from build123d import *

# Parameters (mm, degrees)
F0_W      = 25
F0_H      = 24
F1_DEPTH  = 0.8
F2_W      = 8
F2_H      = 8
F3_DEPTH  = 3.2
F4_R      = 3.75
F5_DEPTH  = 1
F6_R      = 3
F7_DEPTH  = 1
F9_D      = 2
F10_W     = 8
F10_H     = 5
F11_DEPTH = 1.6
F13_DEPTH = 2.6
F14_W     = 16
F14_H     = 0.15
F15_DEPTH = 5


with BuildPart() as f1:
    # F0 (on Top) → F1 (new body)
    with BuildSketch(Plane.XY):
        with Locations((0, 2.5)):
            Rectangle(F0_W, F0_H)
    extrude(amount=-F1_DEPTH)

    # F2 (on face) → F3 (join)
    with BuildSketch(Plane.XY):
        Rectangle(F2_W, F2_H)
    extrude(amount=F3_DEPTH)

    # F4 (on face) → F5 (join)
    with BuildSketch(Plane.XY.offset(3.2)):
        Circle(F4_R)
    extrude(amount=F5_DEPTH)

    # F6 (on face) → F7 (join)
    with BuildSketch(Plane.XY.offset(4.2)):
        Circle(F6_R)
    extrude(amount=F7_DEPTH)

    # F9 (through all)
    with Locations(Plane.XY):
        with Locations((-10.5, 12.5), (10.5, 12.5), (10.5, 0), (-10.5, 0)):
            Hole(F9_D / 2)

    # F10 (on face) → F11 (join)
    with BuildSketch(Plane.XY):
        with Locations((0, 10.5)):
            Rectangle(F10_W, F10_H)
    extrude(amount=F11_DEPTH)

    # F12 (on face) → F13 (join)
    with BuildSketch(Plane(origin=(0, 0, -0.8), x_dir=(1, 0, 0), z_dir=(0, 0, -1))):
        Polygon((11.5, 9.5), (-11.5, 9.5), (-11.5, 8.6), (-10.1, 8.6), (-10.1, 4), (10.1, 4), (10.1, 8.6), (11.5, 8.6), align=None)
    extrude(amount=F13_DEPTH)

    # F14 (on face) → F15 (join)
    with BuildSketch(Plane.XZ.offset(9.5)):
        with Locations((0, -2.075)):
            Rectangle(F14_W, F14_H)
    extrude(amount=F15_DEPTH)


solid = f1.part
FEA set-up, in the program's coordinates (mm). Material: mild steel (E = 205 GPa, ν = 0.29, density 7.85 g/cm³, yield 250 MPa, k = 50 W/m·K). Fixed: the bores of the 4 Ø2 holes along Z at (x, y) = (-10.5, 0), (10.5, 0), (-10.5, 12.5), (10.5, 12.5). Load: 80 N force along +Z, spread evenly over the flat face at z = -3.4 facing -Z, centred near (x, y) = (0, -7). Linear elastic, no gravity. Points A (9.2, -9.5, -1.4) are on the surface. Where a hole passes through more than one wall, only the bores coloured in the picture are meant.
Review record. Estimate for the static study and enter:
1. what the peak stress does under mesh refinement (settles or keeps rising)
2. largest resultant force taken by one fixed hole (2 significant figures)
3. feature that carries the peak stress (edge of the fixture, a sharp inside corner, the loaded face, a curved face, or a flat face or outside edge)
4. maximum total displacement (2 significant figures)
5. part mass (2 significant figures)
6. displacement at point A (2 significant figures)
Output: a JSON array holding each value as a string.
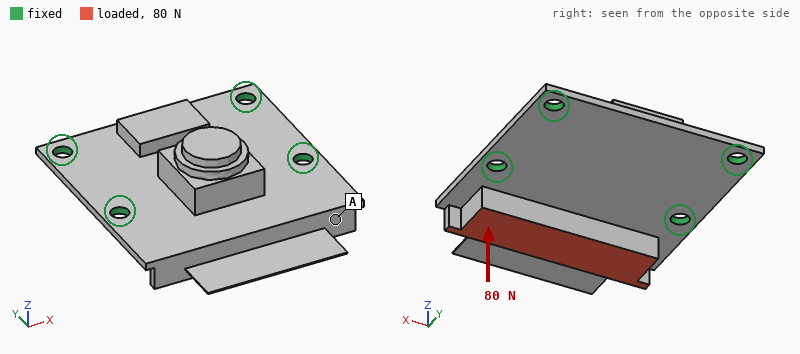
["keeps rising", "50 N", "edge of the fixture", "55 µm", "8.8 g", "34 µm"]
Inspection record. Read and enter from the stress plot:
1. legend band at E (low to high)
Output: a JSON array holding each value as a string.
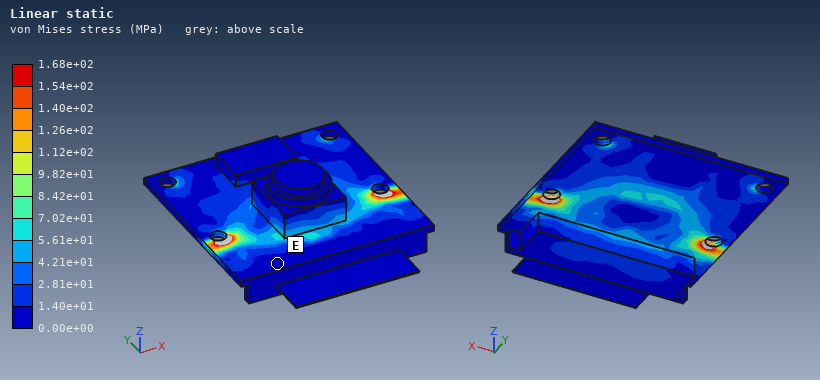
["0.00e+00 to 1.40e+01 MPa"]
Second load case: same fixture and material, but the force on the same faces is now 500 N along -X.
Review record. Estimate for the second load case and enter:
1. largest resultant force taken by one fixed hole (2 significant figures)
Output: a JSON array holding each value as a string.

["280 N"]
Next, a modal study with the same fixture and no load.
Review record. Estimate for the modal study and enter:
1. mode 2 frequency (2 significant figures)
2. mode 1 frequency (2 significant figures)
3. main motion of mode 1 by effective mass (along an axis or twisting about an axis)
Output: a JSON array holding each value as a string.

["5500 Hz", "4200 Hz", "along Z"]
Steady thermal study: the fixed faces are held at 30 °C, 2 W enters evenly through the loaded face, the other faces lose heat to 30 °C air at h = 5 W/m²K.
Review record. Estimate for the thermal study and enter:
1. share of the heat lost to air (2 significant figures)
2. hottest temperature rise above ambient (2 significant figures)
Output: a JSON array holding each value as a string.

["3.0 %", "14 K"]
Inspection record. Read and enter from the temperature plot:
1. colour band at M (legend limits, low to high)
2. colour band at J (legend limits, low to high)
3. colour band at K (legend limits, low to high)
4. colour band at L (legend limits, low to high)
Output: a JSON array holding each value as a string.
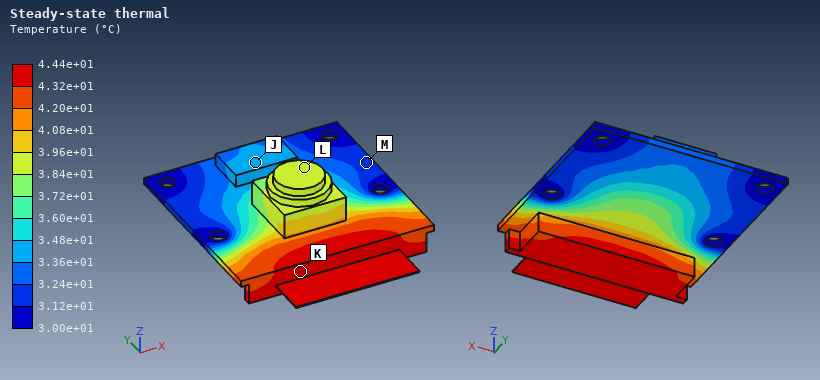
["3.12e+01 to 3.24e+01 °C", "3.36e+01 to 3.48e+01 °C", "4.32e+01 to 4.44e+01 °C", "3.84e+01 to 3.96e+01 °C"]
